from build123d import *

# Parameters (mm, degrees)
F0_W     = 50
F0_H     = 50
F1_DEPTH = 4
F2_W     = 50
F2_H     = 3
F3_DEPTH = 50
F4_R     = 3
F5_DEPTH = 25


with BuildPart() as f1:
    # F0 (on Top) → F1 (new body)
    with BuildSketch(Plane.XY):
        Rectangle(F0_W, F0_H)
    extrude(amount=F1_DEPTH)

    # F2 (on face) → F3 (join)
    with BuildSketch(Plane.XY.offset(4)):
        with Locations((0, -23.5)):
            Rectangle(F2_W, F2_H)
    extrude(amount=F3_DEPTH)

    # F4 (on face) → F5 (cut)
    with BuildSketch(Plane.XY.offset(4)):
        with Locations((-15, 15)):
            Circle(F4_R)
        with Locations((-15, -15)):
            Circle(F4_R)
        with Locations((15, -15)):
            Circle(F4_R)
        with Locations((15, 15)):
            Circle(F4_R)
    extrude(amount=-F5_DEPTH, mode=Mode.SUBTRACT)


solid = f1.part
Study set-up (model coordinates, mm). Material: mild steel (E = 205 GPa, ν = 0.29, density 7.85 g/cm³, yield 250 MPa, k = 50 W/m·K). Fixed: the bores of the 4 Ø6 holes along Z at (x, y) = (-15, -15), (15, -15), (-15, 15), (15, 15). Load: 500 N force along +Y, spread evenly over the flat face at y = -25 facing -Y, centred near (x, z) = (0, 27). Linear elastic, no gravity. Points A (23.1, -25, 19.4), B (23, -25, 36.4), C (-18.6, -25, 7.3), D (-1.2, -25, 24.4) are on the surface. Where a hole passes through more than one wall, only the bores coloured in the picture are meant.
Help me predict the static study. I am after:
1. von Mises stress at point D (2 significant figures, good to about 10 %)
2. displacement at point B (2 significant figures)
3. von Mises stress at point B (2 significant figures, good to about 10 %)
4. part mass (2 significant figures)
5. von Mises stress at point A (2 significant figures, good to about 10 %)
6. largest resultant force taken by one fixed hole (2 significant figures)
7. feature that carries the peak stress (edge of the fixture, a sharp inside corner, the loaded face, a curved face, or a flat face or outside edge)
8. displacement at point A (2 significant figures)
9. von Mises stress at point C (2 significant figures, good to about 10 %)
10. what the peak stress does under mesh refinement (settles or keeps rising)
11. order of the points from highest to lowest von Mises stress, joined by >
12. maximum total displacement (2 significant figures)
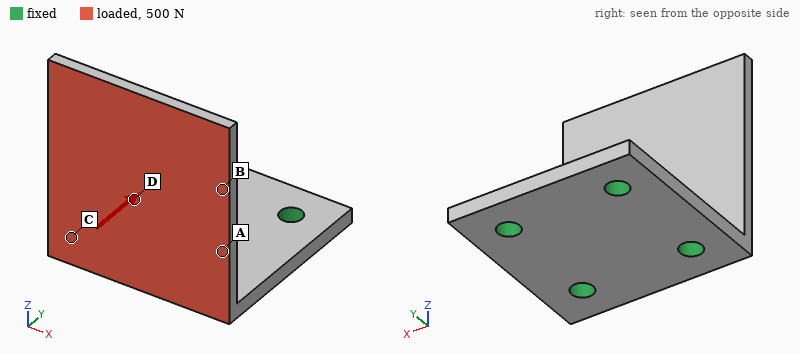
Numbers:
47 MPa
0.23 mm
21 MPa
130 g
77 MPa
220 N
edge of the fixture
0.081 mm
120 MPa
keeps rising
C > A > D > B
0.41 mm
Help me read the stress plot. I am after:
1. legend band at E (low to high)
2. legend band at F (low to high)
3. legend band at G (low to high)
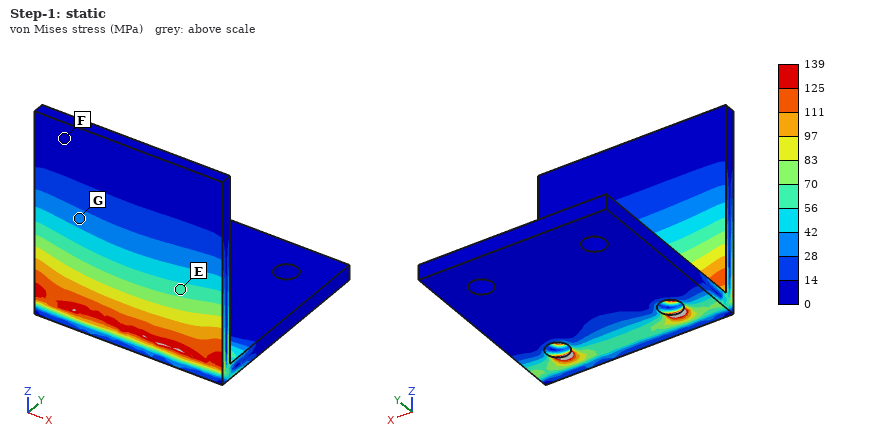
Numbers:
56 to 70 MPa
0 to 14 MPa
28 to 42 MPa
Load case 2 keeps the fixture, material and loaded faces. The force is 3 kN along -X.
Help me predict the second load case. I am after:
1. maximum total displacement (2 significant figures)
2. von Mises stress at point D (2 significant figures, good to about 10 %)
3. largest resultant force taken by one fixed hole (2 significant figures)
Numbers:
65 µm
45 MPa
2.8 kN
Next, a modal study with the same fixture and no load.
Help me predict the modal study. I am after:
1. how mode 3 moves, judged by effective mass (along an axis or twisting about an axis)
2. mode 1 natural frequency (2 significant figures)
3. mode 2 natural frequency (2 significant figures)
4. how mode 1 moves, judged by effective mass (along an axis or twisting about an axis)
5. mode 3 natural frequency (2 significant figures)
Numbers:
along X
870 Hz
2200 Hz
along Y
5000 Hz
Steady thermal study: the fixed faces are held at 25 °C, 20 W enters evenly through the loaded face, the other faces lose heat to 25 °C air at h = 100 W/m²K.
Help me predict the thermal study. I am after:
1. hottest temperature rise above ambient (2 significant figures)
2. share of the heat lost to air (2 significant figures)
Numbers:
38 K
48 %
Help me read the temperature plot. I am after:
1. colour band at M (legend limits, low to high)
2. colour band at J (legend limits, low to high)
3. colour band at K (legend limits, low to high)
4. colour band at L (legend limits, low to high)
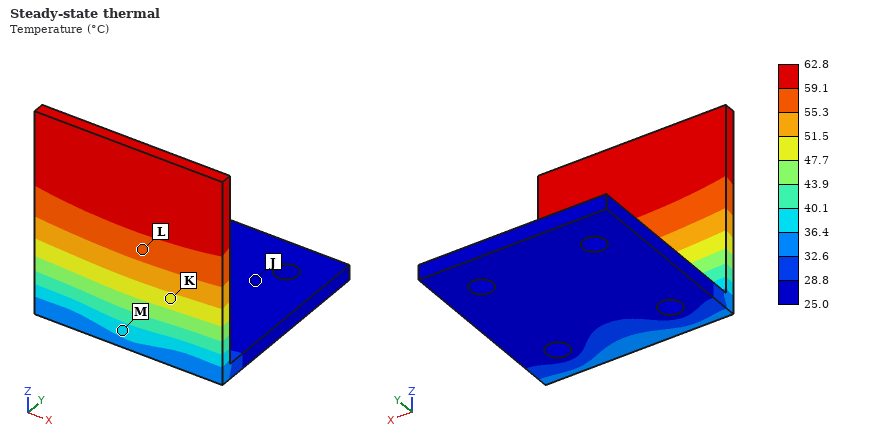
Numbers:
36.4 to 40.1 °C
25.0 to 28.8 °C
47.7 to 51.5 °C
55.3 to 59.1 °C
